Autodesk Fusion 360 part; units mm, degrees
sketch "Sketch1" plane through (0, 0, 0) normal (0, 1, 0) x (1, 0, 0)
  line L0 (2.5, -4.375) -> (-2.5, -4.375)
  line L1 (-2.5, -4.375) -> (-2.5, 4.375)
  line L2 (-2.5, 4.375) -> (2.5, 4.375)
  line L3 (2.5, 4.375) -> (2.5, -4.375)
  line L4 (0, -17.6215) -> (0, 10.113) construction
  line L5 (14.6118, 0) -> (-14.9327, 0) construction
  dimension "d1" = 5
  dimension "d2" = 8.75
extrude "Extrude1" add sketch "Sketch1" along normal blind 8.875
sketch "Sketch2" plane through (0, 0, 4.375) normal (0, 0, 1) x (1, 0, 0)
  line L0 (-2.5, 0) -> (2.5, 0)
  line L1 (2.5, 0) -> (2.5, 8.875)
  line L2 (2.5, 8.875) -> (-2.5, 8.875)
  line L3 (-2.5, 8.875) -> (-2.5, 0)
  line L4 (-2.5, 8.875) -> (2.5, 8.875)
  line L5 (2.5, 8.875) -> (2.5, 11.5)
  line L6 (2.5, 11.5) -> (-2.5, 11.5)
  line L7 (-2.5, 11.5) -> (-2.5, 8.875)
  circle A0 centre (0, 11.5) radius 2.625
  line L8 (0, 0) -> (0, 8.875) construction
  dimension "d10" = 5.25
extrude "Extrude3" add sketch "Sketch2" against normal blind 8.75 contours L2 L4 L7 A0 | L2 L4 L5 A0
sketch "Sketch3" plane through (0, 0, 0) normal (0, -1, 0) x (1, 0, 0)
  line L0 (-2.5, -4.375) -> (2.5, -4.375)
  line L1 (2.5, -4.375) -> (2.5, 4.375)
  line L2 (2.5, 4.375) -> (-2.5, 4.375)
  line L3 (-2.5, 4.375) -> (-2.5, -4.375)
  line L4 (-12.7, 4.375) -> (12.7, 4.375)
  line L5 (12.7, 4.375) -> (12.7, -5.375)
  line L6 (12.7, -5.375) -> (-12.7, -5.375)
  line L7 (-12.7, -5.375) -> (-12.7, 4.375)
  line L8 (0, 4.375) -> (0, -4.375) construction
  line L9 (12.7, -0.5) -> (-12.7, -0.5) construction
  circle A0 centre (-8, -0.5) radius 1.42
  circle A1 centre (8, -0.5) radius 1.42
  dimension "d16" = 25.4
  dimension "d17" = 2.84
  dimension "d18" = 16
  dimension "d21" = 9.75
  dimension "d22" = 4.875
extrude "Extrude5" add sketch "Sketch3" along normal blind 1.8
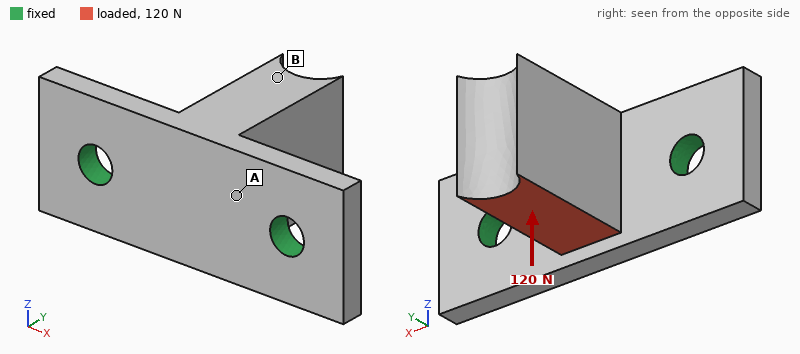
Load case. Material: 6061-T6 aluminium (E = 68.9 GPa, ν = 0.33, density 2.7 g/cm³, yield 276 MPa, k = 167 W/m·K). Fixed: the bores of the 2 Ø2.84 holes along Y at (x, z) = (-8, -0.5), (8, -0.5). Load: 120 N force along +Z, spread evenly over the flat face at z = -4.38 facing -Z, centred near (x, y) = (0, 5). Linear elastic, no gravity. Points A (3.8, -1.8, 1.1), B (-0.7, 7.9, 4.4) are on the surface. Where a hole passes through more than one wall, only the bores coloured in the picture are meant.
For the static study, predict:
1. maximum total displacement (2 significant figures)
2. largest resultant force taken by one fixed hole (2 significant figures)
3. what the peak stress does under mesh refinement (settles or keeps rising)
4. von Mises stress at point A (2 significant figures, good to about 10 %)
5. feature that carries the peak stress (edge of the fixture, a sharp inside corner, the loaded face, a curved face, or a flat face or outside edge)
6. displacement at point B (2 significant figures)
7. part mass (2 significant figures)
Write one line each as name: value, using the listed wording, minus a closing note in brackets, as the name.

maximum total displacement: 37 µm
largest resultant force taken by one fixed hole: 60 N
what the peak stress does under mesh refinement: keeps rising
von Mises stress at point A: 25 MPa
feature that carries the peak stress: edge of the fixture
displacement at point B: 29 µm
part mass: 2.2 g
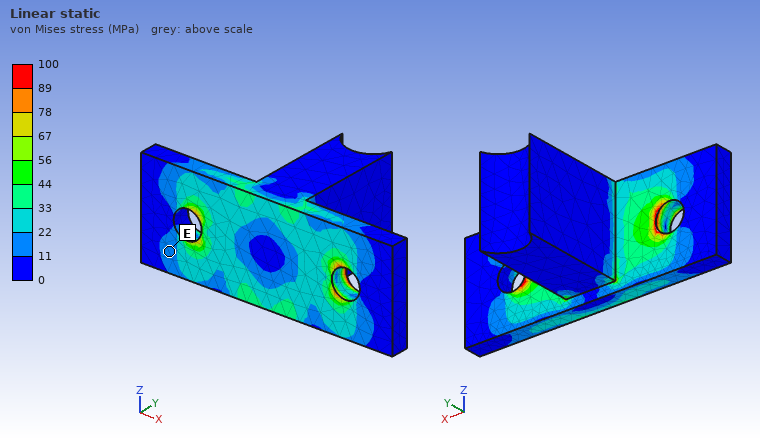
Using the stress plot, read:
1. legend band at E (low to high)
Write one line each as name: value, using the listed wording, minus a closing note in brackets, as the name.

legend band at E: 11 to 22 MPa
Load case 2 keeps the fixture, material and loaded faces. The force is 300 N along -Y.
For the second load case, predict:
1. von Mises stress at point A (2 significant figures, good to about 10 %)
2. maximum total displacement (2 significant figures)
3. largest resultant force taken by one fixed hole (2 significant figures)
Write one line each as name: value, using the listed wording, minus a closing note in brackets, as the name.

von Mises stress at point A: 61 MPa
maximum total displacement: 65 µm
largest resultant force taken by one fixed hole: 160 N
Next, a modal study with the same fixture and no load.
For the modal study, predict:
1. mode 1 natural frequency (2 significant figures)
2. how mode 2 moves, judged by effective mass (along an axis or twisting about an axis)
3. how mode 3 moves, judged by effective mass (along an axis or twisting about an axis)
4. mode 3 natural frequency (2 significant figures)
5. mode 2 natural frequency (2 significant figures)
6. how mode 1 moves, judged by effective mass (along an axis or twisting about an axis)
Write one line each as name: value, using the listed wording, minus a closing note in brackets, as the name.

mode 1 natural frequency: 10 kHz
how mode 2 moves, judged by effective mass: along X
how mode 3 moves, judged by effective mass: along Y
mode 3 natural frequency: 23 kHz
mode 2 natural frequency: 18 kHz
how mode 1 moves, judged by effective mass: along Z
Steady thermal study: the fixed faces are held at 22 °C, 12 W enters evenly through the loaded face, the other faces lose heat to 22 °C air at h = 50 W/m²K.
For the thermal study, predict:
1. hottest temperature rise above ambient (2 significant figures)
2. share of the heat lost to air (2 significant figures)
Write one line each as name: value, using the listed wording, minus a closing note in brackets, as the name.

hottest temperature rise above ambient: 25 K
share of the heat lost to air: 3.2 %
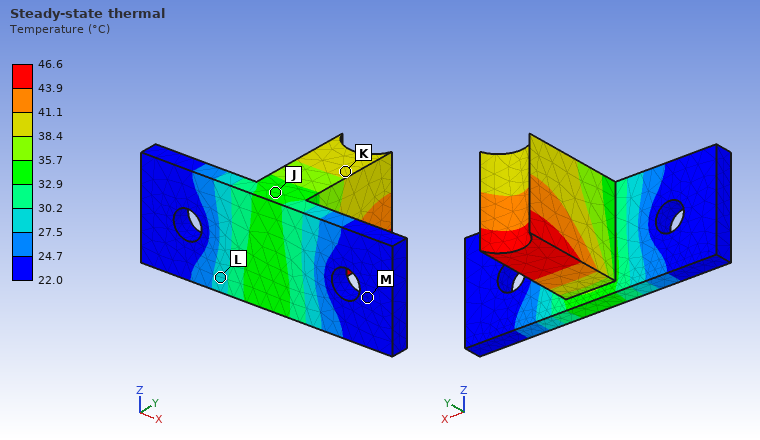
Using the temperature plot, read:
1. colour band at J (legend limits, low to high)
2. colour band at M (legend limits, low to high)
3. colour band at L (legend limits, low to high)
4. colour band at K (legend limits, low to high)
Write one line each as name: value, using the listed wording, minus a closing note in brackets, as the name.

colour band at J: 32.9 to 35.7 °C
colour band at M: 22.0 to 24.7 °C
colour band at L: 27.5 to 30.2 °C
colour band at K: 38.4 to 41.1 °C
